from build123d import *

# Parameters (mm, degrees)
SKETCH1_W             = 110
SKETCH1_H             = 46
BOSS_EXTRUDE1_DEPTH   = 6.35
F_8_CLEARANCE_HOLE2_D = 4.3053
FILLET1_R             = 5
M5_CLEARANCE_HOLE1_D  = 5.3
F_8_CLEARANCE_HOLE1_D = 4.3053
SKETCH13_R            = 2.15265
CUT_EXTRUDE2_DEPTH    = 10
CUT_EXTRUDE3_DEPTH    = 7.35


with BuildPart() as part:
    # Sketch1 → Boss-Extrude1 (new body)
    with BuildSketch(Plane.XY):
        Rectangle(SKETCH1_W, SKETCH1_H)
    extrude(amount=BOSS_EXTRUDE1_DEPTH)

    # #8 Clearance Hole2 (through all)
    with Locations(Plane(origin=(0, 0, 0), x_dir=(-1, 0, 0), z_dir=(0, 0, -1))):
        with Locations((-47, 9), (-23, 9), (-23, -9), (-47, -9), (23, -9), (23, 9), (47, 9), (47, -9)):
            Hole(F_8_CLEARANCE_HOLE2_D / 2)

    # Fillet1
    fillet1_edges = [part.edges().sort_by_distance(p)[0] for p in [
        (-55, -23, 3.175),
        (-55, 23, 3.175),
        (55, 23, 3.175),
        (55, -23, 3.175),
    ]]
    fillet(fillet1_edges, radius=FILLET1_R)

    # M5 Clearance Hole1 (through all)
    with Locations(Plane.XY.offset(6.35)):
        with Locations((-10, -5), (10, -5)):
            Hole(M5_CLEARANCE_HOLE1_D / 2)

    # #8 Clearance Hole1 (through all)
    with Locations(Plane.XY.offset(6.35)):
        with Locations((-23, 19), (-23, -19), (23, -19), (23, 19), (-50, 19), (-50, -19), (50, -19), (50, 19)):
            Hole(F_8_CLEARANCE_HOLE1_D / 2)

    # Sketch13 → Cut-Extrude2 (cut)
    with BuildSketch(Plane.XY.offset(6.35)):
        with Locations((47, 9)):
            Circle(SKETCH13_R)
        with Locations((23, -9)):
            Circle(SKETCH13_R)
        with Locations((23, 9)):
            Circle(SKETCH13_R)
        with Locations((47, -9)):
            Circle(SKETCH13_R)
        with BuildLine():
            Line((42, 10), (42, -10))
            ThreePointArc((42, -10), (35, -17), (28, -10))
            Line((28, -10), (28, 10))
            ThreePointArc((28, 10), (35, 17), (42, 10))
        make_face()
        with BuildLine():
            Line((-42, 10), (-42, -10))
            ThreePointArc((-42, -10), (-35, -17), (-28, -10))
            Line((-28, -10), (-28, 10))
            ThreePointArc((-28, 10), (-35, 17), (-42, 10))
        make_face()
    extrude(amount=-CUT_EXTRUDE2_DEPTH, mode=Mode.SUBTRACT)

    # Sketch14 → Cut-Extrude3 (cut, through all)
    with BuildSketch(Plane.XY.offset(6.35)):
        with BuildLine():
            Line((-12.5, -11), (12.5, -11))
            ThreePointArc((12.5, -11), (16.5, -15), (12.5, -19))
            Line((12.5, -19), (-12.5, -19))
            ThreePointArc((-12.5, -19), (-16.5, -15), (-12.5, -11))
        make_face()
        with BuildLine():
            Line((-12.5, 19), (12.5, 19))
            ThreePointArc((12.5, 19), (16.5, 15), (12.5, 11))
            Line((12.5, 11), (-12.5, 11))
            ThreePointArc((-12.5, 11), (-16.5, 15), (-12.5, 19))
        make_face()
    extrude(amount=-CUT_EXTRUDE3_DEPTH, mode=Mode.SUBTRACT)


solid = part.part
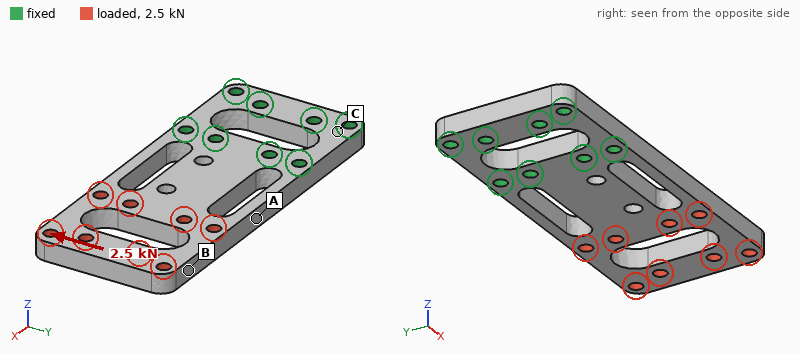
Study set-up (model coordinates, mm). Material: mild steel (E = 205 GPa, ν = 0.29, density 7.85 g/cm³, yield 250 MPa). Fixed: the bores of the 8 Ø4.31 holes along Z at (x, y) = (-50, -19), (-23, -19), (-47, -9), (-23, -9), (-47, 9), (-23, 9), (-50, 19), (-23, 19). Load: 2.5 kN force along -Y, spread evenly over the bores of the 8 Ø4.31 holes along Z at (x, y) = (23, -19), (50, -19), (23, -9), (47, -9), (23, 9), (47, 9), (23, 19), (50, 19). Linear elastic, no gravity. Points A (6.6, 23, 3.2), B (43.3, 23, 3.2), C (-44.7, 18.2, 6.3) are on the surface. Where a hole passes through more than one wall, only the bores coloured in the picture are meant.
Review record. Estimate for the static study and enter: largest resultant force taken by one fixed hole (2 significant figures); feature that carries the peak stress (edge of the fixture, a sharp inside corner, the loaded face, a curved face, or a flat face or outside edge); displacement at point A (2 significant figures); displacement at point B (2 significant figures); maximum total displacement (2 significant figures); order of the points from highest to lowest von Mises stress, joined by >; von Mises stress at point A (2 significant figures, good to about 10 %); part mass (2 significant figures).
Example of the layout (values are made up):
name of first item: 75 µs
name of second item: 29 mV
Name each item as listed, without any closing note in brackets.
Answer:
largest resultant force taken by one fixed hole: 2.6 kN
feature that carries the peak stress: a curved face
displacement at point A: 28 µm
displacement at point B: 66 µm
maximum total displacement: 75 µm
order of the points from highest to lowest von Mises stress, joined by >: A > B > C
von Mises stress at point A: 44 MPa
part mass: 170 g
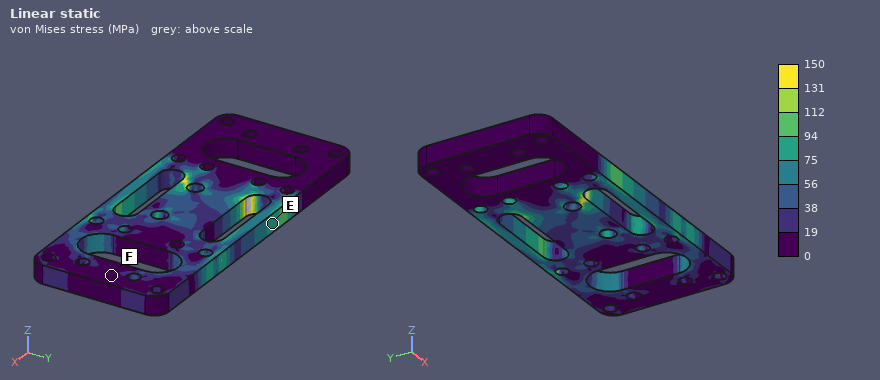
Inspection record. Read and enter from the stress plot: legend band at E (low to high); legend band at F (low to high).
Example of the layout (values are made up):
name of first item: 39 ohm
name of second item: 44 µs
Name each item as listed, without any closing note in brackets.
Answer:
legend band at E: 75 to 94 MPa
legend band at F: 0 to 19 MPa
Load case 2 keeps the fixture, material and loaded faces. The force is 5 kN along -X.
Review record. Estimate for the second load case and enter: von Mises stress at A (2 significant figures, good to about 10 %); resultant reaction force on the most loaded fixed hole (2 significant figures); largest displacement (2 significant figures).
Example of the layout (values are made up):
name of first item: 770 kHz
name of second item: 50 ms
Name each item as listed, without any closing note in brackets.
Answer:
von Mises stress at A: 41 MPa
resultant reaction force on the most loaded fixed hole: 1.4 kN
largest displacement: 17 µm
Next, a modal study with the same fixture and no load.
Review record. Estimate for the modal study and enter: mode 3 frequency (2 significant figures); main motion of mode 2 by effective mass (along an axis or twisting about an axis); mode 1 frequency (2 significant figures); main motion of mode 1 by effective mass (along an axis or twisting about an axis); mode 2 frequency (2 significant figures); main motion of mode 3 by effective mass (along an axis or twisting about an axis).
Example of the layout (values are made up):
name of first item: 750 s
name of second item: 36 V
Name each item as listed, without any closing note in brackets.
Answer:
mode 3 frequency: 4000 Hz
main motion of mode 2 by effective mass: twisting about X
mode 1 frequency: 830 Hz
main motion of mode 1 by effective mass: along Z
mode 2 frequency: 2500 Hz
main motion of mode 3 by effective mass: along Y
